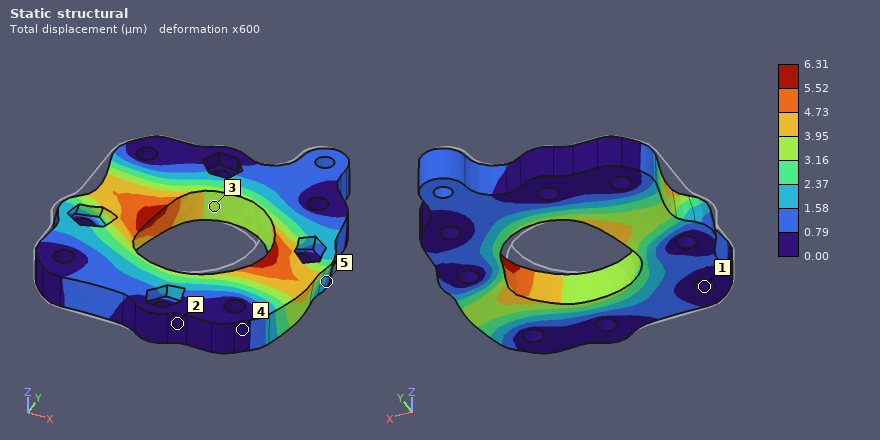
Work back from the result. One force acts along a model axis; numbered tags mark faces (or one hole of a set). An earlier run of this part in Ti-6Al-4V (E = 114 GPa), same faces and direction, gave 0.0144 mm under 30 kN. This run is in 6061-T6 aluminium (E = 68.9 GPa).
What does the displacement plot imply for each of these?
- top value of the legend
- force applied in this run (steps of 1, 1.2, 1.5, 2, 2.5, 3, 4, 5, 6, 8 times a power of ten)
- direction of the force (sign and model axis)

6.31 µm
8 kN
+X
